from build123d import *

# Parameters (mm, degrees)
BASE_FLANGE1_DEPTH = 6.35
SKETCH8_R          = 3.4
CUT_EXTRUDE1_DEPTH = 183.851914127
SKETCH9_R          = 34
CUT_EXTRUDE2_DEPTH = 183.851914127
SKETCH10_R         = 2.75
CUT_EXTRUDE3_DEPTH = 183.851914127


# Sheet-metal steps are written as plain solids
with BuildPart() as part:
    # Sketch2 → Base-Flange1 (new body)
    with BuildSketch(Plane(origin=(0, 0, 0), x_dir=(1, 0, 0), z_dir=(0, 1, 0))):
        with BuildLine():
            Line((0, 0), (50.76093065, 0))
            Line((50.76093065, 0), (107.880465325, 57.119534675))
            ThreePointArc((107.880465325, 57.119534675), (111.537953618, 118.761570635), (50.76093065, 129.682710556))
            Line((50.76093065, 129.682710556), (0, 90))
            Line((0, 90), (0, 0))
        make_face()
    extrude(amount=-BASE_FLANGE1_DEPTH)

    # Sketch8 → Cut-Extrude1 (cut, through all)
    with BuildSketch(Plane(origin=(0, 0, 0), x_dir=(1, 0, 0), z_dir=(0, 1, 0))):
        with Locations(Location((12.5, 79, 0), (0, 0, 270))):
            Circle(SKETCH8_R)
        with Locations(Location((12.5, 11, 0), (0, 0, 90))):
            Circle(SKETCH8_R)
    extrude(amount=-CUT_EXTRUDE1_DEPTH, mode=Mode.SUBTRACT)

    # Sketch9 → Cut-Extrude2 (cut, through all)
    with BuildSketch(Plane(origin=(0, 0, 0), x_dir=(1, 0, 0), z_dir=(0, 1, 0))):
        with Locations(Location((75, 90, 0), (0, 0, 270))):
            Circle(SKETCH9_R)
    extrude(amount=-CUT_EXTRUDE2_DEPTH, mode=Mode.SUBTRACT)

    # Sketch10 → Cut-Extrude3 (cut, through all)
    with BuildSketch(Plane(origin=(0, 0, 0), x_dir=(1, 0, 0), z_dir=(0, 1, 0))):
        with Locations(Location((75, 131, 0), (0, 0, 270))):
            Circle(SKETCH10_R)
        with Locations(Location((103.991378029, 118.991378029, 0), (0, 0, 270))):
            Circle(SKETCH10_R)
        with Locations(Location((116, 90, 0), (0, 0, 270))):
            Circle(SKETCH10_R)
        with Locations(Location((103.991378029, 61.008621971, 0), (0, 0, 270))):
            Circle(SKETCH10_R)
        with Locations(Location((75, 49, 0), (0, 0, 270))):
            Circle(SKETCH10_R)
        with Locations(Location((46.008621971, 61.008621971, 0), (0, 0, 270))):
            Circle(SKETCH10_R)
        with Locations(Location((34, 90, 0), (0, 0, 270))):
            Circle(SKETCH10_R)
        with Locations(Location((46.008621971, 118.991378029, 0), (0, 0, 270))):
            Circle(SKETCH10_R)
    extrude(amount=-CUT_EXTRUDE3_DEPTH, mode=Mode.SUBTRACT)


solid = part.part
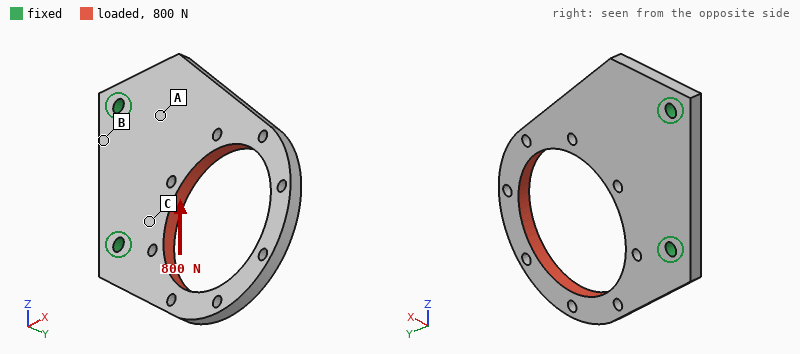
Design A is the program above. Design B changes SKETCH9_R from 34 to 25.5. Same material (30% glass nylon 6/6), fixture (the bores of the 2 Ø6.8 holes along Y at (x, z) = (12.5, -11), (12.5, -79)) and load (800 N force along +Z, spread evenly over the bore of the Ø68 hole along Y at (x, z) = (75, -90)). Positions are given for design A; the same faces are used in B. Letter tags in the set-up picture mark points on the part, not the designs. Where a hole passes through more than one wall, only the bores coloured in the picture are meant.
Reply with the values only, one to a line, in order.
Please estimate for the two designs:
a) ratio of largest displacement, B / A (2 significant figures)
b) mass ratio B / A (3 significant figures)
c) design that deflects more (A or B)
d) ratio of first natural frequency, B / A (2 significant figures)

0.43
1.19
A
0.97
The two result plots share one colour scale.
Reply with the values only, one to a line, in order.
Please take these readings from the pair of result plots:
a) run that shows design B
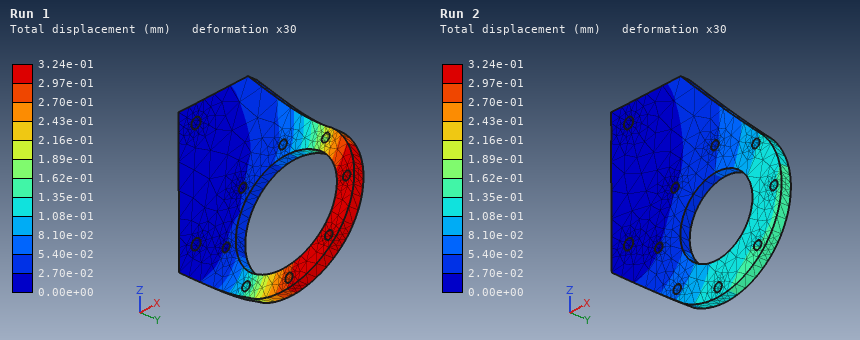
Run 2
